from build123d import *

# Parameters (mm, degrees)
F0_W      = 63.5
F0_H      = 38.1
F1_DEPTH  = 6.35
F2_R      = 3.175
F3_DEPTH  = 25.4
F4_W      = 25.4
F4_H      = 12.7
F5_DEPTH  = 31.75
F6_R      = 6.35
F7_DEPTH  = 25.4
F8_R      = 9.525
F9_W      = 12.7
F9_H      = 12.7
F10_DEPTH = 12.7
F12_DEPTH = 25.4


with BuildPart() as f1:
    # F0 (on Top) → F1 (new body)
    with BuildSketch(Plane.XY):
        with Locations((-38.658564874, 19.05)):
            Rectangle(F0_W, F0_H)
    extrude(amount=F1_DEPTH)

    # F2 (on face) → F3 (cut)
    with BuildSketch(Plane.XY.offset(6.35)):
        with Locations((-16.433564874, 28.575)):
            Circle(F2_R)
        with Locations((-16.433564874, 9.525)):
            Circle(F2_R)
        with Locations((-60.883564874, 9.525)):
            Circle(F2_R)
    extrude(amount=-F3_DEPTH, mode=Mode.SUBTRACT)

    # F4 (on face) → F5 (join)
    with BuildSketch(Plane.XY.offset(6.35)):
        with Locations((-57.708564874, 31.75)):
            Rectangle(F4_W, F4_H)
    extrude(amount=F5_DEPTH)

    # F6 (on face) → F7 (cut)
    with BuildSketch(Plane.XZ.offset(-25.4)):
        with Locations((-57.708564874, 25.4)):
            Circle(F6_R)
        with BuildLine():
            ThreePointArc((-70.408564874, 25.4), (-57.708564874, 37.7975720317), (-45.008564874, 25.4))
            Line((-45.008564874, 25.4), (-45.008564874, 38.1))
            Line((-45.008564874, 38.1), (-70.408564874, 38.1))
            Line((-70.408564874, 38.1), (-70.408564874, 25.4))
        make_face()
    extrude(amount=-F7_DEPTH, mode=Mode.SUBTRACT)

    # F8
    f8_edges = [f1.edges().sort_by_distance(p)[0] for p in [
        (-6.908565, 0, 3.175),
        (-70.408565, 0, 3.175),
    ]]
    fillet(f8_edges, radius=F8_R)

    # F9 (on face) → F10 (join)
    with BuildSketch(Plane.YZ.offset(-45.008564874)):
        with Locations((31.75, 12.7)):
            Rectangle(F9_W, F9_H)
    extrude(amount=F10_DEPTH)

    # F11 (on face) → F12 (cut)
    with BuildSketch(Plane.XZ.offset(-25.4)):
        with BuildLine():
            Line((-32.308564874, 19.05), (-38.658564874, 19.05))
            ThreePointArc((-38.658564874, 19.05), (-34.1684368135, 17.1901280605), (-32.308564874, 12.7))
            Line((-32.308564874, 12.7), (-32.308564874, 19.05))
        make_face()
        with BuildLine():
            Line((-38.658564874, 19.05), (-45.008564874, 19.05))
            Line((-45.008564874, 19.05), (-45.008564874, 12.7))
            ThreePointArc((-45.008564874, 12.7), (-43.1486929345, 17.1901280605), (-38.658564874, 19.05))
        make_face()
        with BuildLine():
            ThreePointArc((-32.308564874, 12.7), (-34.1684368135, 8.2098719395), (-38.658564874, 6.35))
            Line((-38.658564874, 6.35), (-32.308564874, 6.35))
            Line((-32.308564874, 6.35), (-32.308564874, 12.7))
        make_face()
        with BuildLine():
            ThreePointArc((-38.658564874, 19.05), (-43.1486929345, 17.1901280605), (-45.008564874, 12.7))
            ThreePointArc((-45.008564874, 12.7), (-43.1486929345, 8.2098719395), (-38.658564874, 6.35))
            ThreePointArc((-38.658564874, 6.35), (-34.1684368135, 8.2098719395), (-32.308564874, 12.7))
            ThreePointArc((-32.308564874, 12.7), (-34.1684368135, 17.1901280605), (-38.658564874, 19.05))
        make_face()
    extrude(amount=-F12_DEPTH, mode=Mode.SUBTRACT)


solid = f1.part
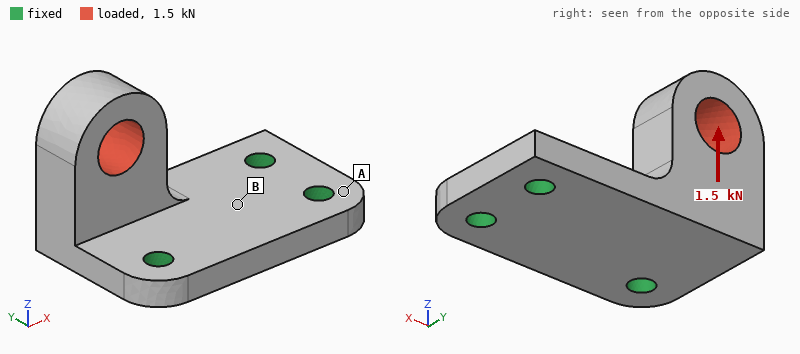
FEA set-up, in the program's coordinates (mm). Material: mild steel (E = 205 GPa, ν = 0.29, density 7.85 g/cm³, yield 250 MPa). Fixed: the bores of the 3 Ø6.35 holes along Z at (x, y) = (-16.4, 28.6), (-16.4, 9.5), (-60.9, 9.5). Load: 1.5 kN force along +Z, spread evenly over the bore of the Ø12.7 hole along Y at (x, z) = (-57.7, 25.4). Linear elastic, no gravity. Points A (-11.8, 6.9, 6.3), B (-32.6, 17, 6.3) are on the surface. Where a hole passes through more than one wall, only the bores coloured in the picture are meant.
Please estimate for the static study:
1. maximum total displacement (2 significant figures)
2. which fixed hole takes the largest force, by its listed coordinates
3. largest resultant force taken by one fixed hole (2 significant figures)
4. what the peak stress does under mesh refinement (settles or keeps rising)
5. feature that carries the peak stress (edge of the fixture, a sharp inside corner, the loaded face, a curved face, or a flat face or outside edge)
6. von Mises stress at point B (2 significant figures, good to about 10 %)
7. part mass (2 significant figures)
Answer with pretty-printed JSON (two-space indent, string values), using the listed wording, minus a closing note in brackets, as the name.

{
  "maximum total displacement": "60 µm",
  "which fixed hole takes the largest force, by its listed coordinates": "(-60.9, 9.5)",
  "largest resultant force taken by one fixed hole": "1.2 kN",
  "what the peak stress does under mesh refinement": "keeps rising",
  "feature that carries the peak stress": "edge of the fixture",
  "von Mises stress at point B": "28 MPa",
  "part mass": "170 g"
}
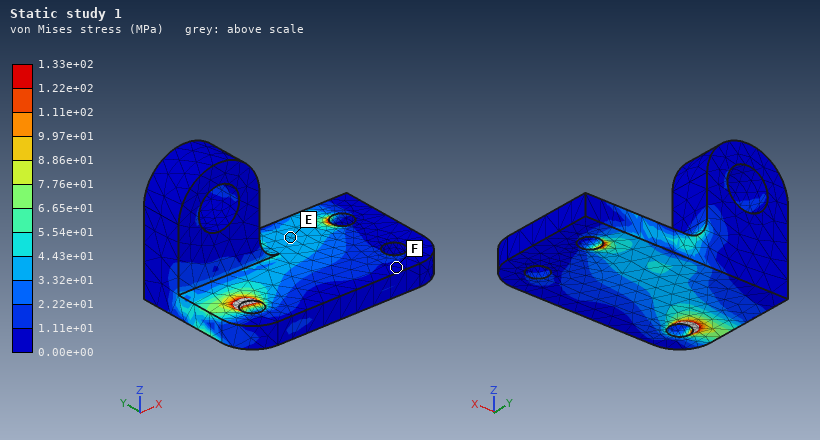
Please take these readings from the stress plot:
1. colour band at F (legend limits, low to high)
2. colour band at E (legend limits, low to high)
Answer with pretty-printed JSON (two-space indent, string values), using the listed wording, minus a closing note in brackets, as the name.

{
  "colour band at F": "0.00e+00 to 1.11e+01 MPa",
  "colour band at E": "3.32e+01 to 4.43e+01 MPa"
}
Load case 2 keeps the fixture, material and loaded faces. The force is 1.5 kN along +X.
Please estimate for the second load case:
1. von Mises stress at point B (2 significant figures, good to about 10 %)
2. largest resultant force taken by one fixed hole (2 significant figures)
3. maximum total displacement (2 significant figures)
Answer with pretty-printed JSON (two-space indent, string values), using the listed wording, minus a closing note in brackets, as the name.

{
  "von Mises stress at point B": "14 MPa",
  "largest resultant force taken by one fixed hole": "970 N",
  "maximum total displacement": "44 µm"
}
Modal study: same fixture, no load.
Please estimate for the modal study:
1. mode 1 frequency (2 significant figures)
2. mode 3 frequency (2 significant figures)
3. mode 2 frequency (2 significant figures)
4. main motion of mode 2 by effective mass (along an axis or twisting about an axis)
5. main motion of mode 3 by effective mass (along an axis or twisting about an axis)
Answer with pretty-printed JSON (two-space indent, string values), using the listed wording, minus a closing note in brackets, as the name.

{
  "mode 1 frequency": "2900 Hz",
  "mode 3 frequency": "8600 Hz",
  "mode 2 frequency": "5800 Hz",
  "main motion of mode 2 by effective mass": "along X",
  "main motion of mode 3 by effective mass": "along Z"
}
